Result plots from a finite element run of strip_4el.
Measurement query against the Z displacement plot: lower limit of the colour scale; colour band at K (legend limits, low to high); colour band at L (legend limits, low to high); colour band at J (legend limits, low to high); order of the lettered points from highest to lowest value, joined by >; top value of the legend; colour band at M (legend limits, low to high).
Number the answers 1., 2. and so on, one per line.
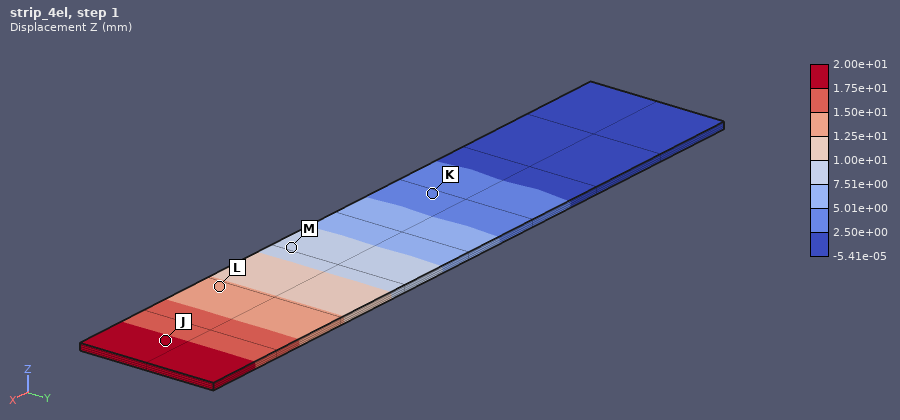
1. -5.41e-05 mm
2. 2.50e+00 to 5.01e+00 mm
3. 1.25e+01 to 1.50e+01 mm
4. 1.75e+01 to 2.00e+01 mm
5. J > L > M > K
6. 2.00e+01 mm
7. 7.51e+00 to 1.00e+01 mm
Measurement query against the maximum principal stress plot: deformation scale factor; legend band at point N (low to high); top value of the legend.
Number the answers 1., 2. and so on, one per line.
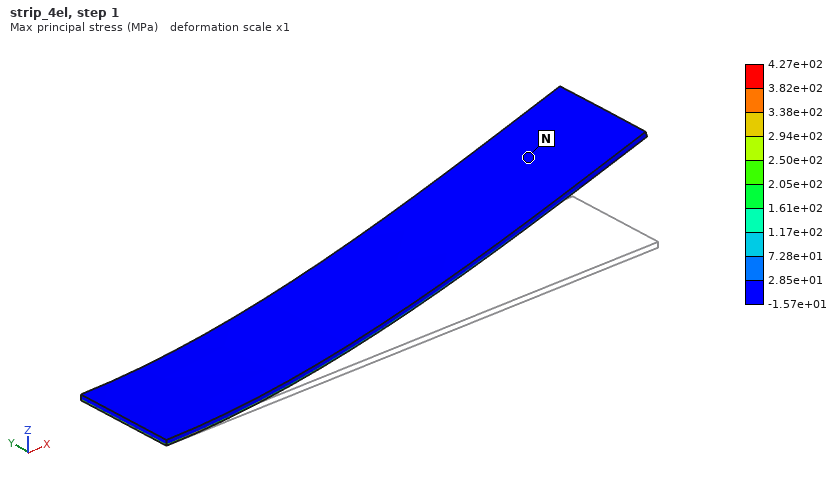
1. 1
2. -1.57e+01 to 2.85e+01 MPa
3. 4.27e+02 MPa
